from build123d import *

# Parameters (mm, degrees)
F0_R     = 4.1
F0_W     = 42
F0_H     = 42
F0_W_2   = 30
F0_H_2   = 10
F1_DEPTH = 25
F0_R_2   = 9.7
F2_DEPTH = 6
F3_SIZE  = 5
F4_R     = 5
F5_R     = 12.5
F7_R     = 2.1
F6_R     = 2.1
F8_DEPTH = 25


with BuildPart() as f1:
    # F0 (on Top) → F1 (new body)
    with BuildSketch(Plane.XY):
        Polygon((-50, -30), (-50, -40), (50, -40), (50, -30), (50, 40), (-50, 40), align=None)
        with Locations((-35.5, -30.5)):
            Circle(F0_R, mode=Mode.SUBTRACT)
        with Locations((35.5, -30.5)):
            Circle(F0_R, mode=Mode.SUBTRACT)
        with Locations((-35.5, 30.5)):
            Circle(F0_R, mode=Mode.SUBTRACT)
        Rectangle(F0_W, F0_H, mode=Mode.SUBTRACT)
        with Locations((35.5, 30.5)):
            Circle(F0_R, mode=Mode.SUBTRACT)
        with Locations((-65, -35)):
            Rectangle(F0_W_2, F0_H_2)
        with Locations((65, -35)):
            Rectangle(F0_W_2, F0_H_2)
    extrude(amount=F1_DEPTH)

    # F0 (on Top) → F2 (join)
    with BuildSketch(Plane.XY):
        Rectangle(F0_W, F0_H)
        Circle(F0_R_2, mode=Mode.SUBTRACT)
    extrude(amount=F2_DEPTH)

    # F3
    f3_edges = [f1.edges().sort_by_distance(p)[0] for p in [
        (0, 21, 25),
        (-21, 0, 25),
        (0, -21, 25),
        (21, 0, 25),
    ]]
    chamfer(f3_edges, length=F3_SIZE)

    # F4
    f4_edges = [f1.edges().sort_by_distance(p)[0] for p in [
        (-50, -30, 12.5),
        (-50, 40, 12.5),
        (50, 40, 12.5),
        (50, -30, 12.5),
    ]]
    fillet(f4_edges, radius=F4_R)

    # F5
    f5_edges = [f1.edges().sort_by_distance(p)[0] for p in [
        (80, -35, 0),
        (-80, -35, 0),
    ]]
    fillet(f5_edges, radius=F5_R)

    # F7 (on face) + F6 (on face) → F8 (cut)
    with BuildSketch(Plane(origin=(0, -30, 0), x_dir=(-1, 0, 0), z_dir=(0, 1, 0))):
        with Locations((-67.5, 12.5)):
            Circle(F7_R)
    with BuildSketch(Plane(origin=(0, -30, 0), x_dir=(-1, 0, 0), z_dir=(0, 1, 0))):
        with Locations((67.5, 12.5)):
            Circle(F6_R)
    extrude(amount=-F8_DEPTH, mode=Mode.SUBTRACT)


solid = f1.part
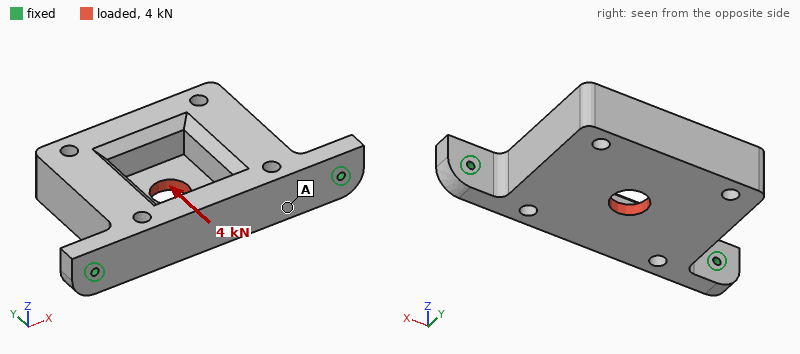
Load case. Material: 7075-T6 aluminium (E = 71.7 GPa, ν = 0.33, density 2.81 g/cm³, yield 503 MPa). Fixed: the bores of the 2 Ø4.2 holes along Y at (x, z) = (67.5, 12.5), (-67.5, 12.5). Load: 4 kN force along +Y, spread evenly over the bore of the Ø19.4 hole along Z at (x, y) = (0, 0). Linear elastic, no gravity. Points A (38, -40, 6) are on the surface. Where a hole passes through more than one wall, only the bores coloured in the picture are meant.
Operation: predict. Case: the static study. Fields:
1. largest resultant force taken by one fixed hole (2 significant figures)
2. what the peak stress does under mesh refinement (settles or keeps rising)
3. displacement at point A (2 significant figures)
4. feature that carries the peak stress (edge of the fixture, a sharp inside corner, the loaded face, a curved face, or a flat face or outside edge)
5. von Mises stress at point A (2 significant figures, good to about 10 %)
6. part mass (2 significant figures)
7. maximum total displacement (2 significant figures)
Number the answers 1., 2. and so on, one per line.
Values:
1. 2.3 kN
2. keeps rising
3. 0.039 mm
4. edge of the fixture
5. 15 MPa
6. 480 g
7. 0.19 mm
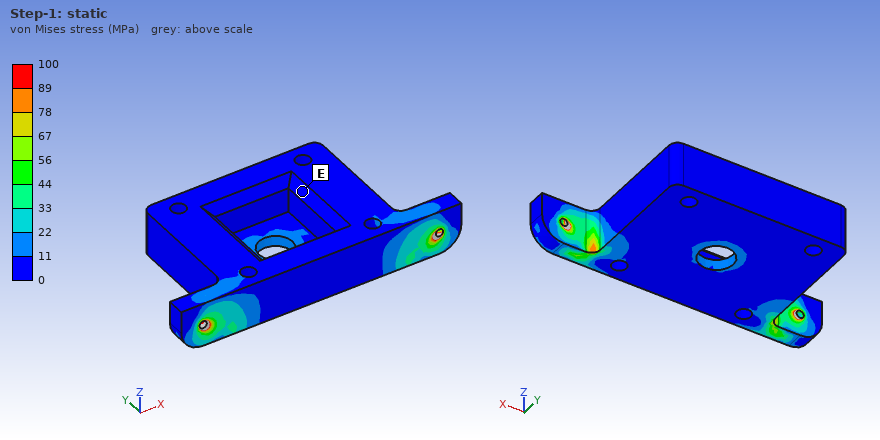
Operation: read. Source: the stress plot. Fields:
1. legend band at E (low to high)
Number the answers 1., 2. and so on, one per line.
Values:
1. 0 to 11 MPa
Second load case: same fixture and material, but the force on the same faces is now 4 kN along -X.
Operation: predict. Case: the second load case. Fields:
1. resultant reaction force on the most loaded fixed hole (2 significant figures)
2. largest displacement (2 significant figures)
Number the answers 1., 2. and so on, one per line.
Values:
1. 2.3 kN
2. 26 µm
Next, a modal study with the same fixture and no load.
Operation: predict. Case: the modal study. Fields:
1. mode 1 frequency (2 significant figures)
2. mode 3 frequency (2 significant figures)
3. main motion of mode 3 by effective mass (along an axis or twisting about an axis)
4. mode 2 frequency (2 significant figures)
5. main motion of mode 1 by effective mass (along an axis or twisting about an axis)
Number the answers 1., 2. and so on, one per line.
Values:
1. 690 Hz
2. 3100 Hz
3. along X
4. 3000 Hz
5. along Z
